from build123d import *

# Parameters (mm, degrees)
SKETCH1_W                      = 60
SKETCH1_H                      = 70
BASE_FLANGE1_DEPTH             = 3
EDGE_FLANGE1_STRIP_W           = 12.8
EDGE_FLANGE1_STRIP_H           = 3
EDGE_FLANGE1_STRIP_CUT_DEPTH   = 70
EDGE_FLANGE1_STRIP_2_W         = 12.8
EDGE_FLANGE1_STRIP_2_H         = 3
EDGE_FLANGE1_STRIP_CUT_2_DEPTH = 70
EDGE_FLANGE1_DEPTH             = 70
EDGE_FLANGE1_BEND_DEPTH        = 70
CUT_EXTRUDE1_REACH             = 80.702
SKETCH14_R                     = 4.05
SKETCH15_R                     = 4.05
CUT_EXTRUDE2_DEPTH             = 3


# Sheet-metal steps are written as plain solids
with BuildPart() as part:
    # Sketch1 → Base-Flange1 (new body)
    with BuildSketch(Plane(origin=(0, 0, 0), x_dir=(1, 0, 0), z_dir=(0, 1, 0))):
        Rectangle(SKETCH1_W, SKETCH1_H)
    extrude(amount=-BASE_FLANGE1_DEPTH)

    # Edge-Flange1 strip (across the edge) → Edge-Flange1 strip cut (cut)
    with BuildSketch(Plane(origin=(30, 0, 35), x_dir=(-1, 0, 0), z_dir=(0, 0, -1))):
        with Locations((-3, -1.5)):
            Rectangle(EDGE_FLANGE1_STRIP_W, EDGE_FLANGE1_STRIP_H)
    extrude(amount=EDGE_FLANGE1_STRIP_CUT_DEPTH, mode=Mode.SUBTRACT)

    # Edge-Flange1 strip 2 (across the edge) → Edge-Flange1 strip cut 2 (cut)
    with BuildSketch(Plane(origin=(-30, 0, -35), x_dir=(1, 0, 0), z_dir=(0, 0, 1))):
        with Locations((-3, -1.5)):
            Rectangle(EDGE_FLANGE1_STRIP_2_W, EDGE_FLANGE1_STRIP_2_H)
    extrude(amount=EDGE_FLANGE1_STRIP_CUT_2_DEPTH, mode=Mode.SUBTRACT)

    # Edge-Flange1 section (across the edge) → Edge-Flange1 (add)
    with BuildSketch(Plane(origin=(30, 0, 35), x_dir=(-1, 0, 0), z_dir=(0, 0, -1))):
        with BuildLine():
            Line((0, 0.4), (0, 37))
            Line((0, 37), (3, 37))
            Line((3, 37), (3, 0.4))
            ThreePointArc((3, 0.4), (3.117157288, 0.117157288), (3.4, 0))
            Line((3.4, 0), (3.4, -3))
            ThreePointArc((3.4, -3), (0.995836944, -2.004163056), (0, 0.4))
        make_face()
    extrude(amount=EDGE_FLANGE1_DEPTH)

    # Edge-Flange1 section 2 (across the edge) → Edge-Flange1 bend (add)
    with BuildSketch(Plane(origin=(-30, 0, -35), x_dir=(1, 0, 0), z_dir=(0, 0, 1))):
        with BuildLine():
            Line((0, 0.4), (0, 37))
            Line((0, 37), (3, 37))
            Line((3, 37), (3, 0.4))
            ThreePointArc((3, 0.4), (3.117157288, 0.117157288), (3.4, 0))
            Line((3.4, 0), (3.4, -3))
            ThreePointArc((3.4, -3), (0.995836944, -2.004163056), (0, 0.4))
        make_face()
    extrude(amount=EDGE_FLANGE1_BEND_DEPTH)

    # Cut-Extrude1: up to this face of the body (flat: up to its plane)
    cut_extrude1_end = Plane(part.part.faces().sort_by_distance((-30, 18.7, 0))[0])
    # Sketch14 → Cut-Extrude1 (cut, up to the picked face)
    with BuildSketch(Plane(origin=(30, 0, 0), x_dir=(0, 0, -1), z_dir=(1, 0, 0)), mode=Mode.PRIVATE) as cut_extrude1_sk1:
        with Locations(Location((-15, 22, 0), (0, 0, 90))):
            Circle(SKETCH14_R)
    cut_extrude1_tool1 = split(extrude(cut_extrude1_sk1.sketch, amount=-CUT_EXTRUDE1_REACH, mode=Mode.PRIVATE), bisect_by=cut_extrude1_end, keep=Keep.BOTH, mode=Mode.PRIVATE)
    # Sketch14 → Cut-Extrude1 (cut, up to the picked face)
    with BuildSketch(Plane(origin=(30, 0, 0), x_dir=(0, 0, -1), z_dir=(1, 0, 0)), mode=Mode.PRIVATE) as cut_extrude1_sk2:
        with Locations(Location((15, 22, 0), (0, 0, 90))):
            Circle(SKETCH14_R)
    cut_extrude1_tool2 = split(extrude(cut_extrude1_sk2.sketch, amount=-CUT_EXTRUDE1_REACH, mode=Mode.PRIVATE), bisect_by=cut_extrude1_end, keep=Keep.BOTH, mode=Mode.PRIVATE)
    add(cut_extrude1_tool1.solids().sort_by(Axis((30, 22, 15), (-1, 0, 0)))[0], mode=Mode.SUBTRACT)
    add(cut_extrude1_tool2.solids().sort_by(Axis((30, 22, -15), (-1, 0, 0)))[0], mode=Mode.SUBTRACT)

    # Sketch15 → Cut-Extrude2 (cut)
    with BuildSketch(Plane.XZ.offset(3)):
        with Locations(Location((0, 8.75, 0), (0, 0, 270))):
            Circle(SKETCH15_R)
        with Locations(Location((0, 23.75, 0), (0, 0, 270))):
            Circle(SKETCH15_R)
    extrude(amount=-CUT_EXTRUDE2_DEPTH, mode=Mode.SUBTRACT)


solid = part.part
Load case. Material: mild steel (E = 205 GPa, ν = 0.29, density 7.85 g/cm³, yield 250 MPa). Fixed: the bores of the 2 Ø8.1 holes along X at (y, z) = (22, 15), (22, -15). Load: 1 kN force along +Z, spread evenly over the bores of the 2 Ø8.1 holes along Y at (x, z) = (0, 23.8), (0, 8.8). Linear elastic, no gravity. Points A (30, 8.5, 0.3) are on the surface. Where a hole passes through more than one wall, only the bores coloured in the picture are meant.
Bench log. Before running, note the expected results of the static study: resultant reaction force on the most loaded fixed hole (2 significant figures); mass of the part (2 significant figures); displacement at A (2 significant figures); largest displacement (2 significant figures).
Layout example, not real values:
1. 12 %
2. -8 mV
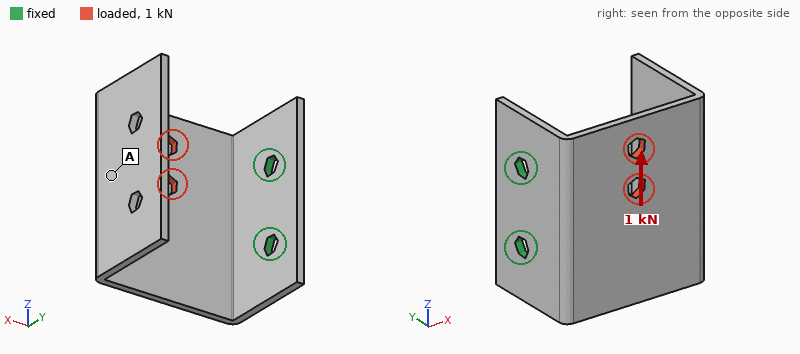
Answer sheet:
1. 1.0 kN
2. 210 g
3. 0.27 mm
4. 0.39 mm
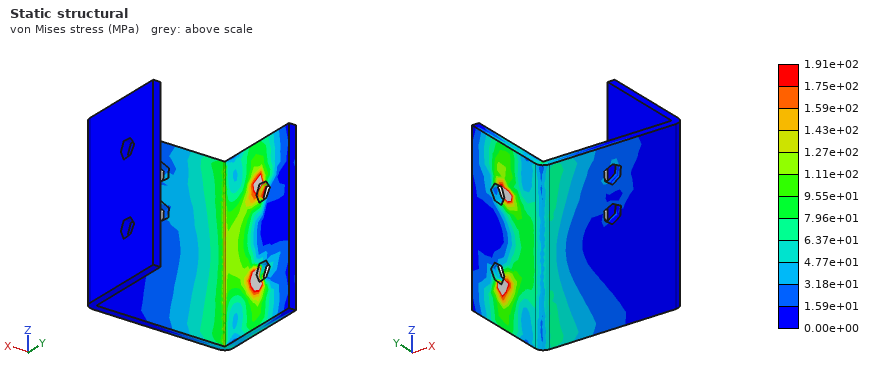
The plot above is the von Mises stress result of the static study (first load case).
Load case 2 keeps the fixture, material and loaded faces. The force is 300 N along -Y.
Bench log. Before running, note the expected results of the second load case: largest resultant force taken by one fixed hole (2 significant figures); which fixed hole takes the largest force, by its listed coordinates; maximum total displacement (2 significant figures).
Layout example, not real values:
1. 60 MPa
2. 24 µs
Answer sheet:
1. 280 N
2. (22, 15)
3. 0.62 mm
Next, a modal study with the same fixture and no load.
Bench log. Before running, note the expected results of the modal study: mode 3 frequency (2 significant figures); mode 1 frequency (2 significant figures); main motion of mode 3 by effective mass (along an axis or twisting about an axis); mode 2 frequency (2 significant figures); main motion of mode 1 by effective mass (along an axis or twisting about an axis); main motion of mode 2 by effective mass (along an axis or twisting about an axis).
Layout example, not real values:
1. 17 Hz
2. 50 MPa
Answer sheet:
1. 880 Hz
2. 260 Hz
3. along X
4. 500 Hz
5. along Y
6. along Z
